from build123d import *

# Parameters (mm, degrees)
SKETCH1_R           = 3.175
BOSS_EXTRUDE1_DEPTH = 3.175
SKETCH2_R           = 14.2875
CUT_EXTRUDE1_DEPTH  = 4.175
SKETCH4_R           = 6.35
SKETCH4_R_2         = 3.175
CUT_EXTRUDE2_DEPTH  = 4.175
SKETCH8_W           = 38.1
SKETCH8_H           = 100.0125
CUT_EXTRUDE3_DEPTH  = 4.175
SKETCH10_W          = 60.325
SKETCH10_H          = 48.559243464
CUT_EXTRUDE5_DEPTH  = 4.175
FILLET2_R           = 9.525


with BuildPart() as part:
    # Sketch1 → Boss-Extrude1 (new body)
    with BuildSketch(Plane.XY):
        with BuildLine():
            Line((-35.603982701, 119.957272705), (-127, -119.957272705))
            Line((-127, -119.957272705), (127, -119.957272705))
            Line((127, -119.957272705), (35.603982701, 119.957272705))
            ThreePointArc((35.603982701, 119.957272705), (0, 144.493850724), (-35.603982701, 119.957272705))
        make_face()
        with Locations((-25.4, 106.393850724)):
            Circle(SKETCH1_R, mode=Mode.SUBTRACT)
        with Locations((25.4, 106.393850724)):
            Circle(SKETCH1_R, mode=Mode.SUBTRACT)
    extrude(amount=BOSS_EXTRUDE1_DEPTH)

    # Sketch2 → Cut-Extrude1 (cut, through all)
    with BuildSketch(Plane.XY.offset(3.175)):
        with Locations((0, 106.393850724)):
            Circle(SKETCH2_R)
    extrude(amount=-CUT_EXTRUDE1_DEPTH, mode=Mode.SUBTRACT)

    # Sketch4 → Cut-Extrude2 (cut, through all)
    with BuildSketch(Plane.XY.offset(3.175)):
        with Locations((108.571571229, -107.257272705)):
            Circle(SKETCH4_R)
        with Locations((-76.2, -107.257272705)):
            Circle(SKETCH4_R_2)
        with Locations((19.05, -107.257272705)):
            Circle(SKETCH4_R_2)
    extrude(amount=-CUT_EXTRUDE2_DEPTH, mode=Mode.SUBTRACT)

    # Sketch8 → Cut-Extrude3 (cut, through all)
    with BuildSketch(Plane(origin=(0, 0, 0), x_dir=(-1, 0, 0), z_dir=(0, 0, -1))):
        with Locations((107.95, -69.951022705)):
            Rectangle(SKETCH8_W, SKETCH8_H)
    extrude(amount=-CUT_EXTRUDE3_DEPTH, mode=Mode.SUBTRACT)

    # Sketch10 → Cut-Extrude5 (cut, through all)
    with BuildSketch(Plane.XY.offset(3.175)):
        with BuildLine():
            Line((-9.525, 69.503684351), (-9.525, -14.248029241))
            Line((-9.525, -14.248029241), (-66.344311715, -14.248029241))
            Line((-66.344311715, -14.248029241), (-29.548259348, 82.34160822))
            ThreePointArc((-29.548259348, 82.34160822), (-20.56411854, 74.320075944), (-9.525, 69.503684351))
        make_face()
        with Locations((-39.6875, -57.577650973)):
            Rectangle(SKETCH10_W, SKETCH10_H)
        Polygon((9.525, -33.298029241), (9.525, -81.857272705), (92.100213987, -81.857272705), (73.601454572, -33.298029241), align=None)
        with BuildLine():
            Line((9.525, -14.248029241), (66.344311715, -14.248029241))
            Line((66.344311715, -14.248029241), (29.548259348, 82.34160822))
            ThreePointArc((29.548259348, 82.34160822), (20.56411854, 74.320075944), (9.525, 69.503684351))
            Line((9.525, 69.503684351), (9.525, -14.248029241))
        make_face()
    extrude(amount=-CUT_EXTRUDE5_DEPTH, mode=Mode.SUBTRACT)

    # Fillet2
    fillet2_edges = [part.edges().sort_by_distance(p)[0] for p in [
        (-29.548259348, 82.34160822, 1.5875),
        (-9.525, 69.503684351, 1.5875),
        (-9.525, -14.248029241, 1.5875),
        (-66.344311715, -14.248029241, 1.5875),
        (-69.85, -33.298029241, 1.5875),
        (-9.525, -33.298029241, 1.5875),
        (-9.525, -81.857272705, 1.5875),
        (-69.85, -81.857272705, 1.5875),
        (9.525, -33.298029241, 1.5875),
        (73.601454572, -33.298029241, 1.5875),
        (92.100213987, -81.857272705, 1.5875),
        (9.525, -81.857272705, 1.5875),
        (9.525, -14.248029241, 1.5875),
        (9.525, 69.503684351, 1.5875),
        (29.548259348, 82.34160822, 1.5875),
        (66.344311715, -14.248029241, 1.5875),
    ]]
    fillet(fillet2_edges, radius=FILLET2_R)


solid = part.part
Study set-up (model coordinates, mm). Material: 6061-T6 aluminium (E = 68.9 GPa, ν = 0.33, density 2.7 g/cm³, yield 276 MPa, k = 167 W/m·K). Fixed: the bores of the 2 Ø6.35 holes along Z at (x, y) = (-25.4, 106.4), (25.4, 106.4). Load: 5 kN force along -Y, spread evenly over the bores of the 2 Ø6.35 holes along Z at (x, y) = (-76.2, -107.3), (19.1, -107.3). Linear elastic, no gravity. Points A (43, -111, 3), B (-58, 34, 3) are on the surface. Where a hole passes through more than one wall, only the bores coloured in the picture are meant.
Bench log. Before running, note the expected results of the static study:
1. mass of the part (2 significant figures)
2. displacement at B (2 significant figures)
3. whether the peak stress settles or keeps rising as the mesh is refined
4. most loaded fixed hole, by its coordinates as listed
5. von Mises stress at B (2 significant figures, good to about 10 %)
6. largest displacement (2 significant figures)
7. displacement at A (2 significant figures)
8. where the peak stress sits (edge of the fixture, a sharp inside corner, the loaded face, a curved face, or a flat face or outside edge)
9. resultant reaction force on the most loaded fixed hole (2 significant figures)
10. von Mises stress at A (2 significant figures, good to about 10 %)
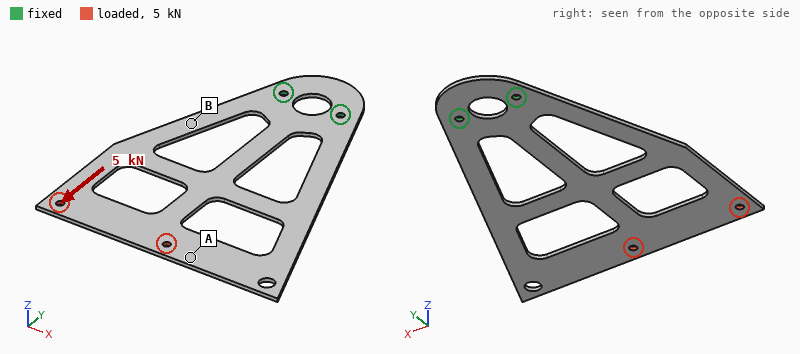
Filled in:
210 g
0.23 mm
keeps rising
(-25.4, 106.4)
45 MPa
0.68 mm
0.59 mm
edge of the fixture
5.1 kN
11 MPa
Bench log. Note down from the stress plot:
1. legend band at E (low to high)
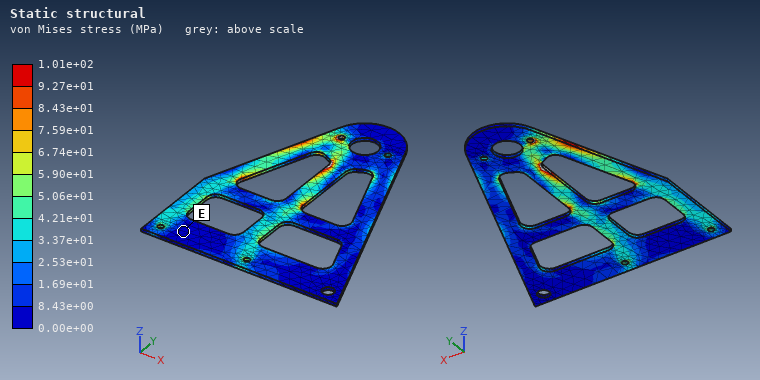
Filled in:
0.00e+00 to 8.43e+00 MPa
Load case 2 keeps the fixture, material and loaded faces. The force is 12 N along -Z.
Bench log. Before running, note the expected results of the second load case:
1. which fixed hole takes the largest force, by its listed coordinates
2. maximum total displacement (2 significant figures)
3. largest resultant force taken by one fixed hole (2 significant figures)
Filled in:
(-25.4, 106.4)
3.9 mm
10 N
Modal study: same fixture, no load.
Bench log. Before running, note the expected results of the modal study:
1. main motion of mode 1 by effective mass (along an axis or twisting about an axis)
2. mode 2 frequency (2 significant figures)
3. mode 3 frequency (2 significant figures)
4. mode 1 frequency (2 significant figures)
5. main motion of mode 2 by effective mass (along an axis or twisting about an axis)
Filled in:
along Z
86 Hz
240 Hz
34 Hz
twisting about Y
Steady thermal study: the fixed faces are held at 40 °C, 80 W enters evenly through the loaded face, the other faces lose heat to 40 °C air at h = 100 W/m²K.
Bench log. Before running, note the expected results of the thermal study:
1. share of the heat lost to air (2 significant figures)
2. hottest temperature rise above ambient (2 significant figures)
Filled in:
99 %
86 K
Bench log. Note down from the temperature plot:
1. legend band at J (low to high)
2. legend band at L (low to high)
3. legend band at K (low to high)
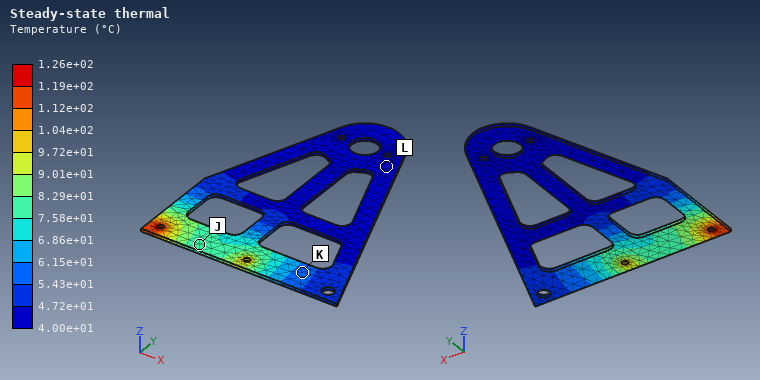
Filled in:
7.58e+01 to 8.29e+01 °C
4.00e+01 to 4.72e+01 °C
5.43e+01 to 6.15e+01 °C
